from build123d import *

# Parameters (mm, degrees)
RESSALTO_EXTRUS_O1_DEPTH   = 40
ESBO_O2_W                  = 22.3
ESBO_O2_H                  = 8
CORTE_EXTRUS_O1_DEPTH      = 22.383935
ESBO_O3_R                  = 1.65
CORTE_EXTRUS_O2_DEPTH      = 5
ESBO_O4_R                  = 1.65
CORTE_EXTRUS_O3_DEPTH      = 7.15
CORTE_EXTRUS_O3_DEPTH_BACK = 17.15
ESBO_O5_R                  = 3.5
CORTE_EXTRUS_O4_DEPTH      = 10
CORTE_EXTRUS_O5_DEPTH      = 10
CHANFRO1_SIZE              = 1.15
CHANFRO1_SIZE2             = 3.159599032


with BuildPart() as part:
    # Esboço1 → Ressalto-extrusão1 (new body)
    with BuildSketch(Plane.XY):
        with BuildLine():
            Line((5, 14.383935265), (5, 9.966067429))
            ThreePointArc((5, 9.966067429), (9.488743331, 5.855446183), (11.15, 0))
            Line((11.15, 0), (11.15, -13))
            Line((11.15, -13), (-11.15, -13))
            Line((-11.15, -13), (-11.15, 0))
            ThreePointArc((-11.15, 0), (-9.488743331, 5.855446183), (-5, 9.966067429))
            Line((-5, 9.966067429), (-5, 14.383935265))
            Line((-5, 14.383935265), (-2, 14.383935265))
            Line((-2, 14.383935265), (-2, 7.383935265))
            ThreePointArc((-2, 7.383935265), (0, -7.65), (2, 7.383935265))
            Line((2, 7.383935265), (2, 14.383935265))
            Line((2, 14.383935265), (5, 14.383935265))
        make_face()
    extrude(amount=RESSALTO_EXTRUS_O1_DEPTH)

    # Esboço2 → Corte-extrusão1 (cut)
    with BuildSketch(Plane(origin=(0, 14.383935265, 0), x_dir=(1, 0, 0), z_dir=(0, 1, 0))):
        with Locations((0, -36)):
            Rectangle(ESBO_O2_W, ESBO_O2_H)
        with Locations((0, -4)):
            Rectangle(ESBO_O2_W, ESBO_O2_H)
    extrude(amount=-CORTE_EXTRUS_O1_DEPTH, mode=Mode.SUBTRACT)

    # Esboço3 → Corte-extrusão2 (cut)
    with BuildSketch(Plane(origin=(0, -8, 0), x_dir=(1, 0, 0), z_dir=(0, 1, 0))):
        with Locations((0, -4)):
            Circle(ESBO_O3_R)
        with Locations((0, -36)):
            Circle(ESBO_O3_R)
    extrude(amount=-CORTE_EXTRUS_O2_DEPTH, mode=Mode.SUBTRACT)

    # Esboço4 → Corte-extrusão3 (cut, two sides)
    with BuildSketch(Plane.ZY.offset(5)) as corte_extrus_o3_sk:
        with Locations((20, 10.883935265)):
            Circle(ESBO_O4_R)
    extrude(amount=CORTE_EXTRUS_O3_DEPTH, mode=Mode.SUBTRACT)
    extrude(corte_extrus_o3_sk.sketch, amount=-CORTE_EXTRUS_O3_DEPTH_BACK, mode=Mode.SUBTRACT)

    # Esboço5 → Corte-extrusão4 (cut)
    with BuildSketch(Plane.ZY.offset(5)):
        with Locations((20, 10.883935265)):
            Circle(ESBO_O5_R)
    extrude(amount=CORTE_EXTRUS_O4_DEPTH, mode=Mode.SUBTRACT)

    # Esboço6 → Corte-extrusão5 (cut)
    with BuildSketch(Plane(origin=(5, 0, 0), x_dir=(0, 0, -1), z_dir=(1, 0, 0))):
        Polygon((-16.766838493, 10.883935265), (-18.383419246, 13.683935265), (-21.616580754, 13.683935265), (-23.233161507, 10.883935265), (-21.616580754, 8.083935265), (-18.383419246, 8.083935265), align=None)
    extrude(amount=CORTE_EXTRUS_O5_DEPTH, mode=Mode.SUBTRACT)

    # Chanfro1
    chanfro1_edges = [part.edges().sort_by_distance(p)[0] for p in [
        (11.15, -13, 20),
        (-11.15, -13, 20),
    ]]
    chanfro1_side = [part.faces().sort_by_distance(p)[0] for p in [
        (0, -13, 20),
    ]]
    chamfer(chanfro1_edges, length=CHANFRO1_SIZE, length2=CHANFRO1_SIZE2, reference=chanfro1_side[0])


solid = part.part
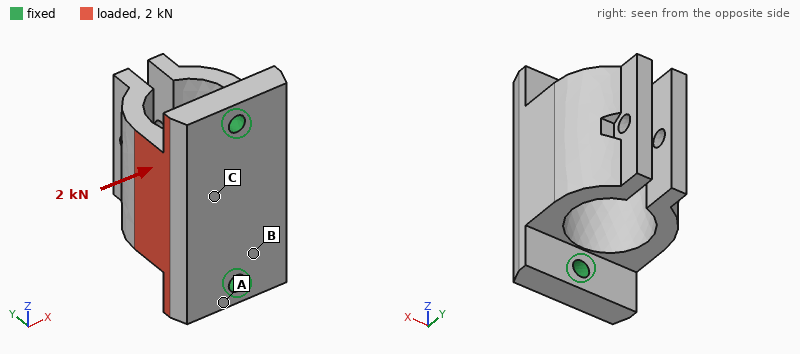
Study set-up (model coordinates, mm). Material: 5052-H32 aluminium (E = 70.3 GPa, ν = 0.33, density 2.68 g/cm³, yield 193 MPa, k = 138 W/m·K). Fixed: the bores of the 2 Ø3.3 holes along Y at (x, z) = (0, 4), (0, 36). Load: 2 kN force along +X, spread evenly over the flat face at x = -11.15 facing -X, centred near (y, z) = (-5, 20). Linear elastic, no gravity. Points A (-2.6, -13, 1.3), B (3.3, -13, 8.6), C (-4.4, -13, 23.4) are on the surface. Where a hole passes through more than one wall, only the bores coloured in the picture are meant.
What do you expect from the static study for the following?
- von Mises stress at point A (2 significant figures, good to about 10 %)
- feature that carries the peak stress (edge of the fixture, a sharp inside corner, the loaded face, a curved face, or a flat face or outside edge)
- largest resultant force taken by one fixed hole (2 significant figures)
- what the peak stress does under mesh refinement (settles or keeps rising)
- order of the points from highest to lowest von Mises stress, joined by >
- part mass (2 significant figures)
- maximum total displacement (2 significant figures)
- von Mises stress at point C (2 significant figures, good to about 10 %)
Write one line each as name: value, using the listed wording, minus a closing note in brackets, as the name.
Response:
von Mises stress at point A: 44 MPa
feature that carries the peak stress: edge of the fixture
largest resultant force taken by one fixed hole: 1.0 kN
what the peak stress does under mesh refinement: keeps rising
order of the points from highest to lowest von Mises stress, joined by >: A > C > B
part mass: 24 g
maximum total displacement: 93 µm
von Mises stress at point C: 24 MPa
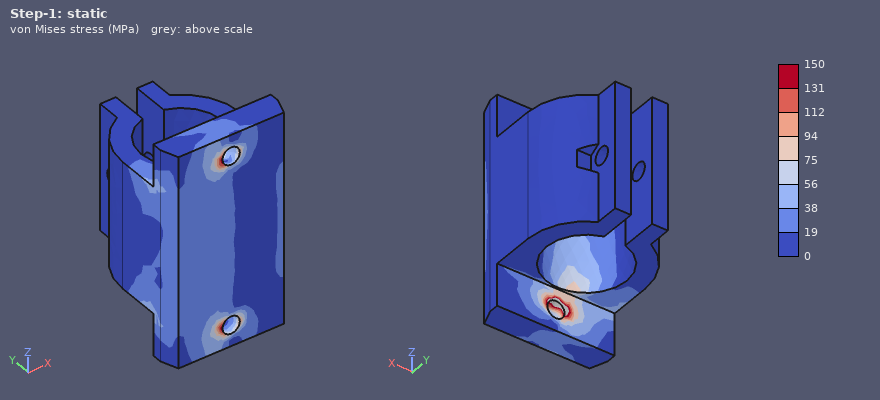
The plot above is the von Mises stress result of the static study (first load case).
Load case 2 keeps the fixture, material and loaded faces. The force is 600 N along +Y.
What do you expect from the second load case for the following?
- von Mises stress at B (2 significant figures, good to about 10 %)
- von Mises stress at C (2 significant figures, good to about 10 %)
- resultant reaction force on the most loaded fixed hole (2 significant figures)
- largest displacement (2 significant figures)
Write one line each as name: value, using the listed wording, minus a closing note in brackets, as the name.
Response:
von Mises stress at B: 12 MPa
von Mises stress at C: 12 MPa
resultant reaction force on the most loaded fixed hole: 310 N
largest displacement: 45 µm
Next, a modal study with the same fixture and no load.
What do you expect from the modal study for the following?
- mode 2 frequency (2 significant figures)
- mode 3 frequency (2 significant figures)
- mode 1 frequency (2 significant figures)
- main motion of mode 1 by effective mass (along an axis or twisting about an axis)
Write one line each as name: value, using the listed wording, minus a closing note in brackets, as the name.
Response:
mode 2 frequency: 6300 Hz
mode 3 frequency: 11 kHz
mode 1 frequency: 5000 Hz
main motion of mode 1 by effective mass: along X
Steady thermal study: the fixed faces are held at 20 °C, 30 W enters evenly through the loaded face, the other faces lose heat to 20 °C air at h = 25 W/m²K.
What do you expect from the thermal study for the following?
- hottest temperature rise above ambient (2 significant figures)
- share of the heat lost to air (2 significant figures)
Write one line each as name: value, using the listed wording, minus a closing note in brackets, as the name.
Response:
hottest temperature rise above ambient: 21 K
share of the heat lost to air: 3.8 %
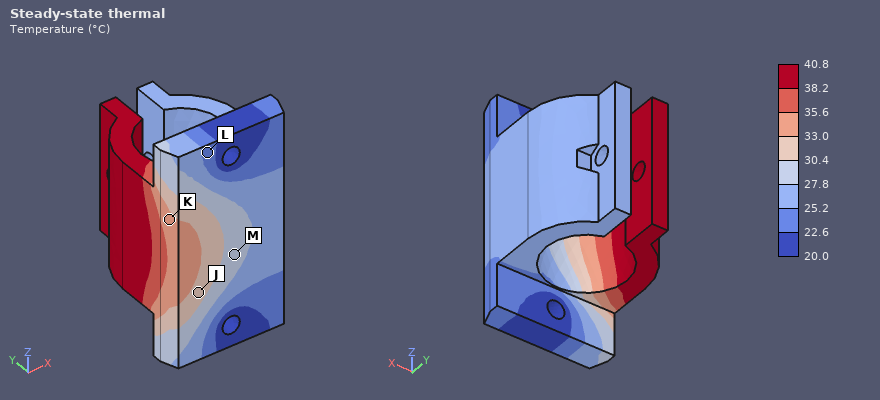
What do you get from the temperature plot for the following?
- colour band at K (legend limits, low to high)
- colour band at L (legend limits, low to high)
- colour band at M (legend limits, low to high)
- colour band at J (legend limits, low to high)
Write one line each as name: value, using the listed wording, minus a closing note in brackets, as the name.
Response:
colour band at K: 33.0 to 35.6 °C
colour band at L: 22.6 to 25.2 °C
colour band at M: 27.8 to 30.4 °C
colour band at J: 30.4 to 33.0 °C
